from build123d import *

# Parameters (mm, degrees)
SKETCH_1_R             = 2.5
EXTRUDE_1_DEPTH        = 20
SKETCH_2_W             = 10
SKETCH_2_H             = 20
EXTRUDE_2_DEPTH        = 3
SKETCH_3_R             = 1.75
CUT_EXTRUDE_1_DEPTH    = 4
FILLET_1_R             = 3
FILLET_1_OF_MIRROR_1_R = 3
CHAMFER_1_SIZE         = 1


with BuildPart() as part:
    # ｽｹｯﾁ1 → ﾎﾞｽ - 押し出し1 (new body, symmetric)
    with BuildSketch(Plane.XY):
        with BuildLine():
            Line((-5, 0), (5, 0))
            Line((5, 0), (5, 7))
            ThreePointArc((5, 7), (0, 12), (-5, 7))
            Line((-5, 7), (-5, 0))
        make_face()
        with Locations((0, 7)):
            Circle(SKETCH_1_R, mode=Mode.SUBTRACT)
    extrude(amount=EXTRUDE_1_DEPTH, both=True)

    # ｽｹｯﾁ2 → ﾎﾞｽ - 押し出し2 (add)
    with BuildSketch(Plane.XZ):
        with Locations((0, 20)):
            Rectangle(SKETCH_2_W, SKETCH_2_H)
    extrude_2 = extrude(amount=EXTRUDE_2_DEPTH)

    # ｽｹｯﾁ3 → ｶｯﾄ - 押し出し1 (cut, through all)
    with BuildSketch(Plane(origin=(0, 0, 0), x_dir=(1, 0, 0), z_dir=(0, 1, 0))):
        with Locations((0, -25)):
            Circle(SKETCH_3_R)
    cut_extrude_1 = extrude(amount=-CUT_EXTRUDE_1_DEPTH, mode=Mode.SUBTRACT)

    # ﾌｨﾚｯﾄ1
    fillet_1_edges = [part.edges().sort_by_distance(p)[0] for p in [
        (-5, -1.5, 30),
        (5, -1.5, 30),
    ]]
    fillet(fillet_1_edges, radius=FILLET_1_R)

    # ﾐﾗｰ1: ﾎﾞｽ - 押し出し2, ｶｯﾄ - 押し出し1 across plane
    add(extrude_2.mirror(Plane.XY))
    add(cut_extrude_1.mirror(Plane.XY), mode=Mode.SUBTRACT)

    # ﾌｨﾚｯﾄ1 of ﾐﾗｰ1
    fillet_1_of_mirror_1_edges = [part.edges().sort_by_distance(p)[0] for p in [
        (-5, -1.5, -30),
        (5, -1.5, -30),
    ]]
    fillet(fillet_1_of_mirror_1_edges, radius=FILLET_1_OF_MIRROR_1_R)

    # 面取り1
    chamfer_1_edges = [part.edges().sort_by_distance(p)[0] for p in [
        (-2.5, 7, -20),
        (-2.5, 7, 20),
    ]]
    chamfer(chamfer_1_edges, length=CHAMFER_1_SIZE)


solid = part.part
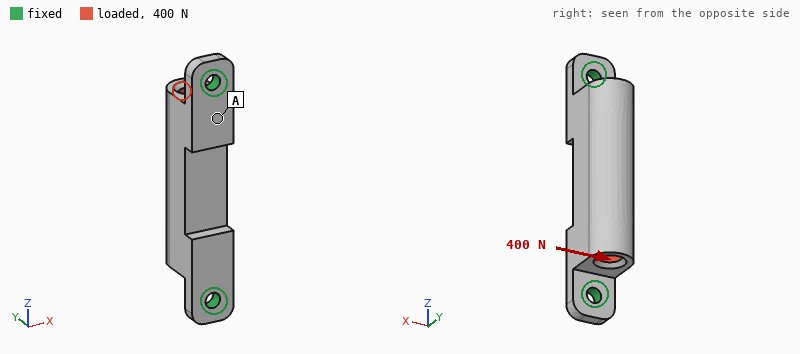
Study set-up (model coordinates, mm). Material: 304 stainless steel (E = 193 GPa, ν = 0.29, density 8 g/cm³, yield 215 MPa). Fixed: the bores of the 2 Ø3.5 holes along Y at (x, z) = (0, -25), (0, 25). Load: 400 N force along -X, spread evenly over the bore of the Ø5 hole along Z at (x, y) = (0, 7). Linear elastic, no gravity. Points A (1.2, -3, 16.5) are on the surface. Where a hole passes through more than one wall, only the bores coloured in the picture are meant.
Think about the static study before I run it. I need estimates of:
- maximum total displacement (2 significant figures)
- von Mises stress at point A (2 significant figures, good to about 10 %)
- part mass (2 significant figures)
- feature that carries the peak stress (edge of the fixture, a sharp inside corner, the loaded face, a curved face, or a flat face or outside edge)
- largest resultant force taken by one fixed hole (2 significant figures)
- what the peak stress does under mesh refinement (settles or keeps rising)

20 µm
14 MPa
37 g
edge of the fixture
200 N
keeps rising
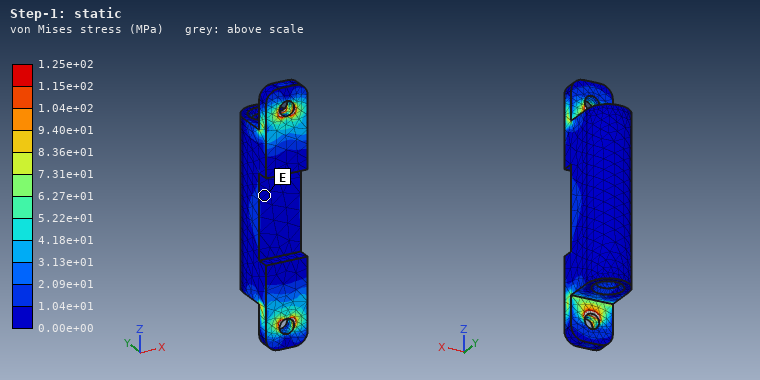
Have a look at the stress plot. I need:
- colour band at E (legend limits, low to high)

0.00e+00 to 1.04e+01 MPa
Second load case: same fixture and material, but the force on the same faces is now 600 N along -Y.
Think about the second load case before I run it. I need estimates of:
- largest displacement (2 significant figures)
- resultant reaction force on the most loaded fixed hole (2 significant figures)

3.7 µm
430 N
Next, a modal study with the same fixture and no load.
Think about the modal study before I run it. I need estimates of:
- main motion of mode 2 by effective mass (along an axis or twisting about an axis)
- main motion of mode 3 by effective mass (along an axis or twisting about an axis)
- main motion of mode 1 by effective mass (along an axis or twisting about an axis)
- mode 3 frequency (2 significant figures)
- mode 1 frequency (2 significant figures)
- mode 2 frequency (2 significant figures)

along Y
along X
along X
17 kHz
5500 Hz
12 kHz
